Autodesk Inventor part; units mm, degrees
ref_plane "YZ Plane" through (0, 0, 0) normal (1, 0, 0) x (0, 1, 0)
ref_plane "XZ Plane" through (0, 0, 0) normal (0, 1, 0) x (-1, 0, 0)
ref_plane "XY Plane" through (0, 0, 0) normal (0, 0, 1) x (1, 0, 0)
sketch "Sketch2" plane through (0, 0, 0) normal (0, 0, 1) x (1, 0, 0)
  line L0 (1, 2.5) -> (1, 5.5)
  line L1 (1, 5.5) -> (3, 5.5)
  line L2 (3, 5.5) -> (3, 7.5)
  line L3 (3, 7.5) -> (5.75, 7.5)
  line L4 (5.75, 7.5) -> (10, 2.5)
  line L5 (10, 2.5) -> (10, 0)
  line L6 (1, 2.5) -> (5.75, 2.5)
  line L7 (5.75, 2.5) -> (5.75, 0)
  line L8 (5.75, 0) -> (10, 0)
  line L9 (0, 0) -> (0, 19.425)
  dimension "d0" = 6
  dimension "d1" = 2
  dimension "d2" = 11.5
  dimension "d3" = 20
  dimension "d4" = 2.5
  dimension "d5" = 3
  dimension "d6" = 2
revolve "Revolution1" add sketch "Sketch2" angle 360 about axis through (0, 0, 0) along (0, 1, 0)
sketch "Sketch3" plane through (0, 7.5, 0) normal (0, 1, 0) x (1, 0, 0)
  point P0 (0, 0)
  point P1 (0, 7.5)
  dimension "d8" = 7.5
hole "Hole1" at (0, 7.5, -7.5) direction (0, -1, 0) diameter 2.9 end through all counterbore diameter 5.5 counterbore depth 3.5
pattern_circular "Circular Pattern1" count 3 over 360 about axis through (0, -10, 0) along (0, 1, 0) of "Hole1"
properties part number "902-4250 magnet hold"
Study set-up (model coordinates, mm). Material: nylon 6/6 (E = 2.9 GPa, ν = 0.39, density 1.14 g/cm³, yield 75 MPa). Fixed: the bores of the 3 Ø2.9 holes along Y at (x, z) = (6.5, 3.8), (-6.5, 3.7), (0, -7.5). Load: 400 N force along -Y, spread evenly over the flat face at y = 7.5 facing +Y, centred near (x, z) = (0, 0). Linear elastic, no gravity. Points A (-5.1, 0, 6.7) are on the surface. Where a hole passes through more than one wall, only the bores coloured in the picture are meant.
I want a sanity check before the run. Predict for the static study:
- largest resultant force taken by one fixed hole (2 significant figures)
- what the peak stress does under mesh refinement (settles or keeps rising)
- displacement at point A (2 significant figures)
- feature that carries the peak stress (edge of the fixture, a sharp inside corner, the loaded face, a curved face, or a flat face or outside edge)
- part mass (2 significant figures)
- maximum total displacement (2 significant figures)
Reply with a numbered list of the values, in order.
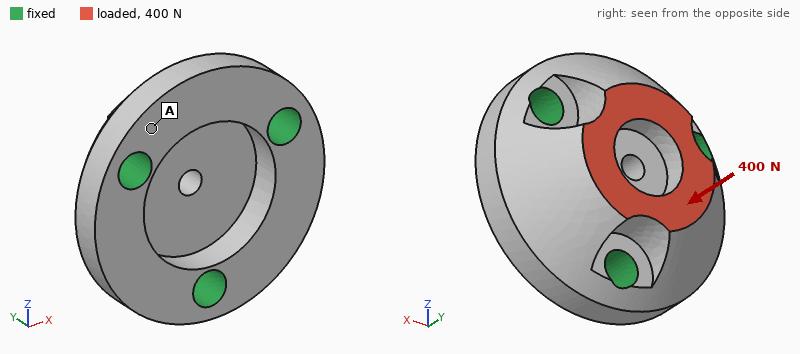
1. 140 N
2. keeps rising
3. 7.5 µm
4. edge of the fixture
5. 1.5 g
6. 28 µm
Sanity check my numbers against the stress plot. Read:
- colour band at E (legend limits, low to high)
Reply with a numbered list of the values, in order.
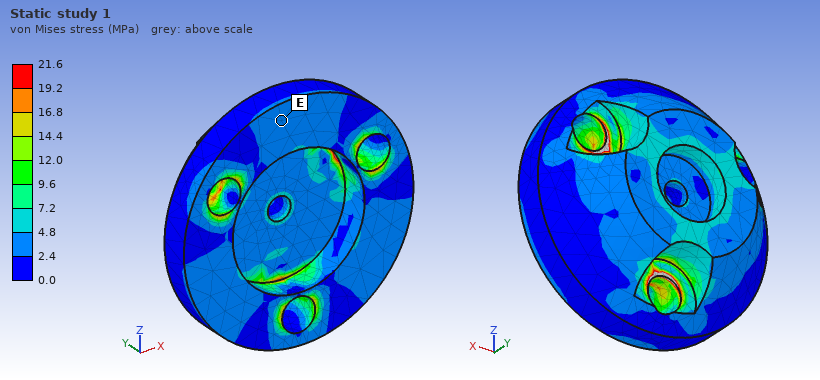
1. 2.4 to 4.8 MPa
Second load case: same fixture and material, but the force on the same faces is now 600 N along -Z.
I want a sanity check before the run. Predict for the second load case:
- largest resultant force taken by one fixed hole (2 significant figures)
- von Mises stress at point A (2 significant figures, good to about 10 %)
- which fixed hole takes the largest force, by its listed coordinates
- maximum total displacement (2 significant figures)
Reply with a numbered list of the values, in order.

1. 320 N
2. 5.8 MPa
3. (0, -7.5)
4. 83 µm
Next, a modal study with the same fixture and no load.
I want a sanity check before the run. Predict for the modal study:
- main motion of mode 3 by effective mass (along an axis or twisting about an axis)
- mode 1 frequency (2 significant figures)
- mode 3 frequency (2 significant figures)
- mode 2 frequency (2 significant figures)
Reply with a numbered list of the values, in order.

1. along Y
2. 21 kHz
3. 22 kHz
4. 21 kHz
